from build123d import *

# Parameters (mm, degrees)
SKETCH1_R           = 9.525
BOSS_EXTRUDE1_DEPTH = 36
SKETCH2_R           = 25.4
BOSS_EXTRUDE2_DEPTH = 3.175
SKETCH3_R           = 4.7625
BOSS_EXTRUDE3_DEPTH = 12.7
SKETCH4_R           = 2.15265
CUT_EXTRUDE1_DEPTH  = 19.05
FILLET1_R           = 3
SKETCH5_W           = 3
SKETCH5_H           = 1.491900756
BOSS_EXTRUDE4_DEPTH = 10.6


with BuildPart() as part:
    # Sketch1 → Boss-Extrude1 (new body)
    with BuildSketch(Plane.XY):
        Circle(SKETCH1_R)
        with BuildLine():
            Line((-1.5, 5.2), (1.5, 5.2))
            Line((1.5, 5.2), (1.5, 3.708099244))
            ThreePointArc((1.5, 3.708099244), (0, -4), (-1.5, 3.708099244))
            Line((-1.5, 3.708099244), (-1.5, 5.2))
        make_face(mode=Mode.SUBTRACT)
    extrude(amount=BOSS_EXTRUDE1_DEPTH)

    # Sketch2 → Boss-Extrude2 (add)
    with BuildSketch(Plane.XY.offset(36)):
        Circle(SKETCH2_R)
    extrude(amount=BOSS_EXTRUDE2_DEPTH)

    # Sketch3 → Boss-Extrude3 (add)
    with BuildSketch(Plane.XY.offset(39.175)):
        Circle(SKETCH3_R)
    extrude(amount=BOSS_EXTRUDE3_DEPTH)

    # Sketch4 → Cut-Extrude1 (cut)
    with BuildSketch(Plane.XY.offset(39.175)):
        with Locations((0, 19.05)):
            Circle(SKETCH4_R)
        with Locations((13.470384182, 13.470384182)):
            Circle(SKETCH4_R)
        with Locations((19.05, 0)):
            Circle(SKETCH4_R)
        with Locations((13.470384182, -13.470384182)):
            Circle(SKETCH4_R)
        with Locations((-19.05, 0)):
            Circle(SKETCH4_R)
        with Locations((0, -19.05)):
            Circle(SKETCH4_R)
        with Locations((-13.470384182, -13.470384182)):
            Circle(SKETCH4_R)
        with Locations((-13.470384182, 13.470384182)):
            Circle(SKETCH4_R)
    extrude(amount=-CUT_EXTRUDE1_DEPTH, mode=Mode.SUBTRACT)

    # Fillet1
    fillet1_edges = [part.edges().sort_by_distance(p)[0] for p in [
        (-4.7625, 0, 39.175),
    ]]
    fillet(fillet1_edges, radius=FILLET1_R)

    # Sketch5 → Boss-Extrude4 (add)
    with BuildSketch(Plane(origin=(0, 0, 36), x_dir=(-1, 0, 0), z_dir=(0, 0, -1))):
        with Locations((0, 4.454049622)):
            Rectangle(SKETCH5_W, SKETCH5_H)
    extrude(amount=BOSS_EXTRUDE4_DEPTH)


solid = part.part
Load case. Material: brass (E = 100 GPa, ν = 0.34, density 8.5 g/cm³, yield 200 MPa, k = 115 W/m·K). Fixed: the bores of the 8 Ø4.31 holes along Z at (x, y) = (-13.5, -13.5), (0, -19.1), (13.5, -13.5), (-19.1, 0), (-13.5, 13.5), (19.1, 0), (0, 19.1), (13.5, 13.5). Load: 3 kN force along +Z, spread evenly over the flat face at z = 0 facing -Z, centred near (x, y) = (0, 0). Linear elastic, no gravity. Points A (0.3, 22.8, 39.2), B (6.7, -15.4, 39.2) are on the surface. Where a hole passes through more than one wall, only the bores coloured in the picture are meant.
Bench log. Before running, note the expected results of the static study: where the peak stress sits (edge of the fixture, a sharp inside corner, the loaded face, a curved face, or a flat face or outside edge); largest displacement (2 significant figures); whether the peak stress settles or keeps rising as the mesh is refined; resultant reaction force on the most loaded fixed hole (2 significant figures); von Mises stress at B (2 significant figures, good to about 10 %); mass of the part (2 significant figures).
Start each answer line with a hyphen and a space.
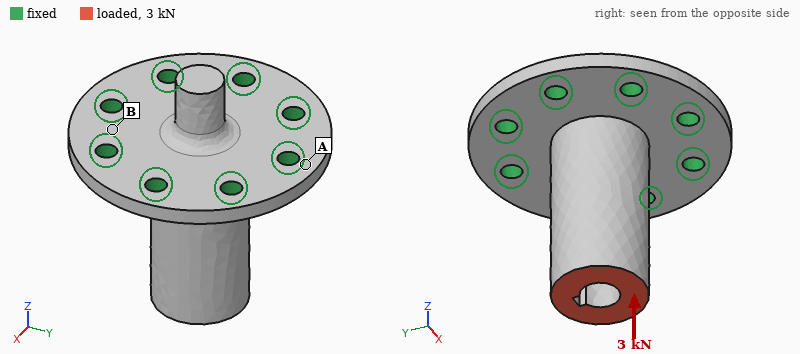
- edge of the fixture
- 19 µm
- keeps rising
- 410 N
- 34 MPa
- 130 g
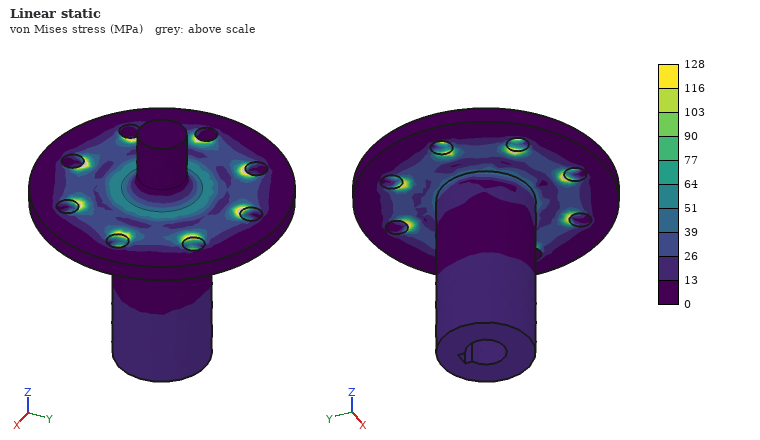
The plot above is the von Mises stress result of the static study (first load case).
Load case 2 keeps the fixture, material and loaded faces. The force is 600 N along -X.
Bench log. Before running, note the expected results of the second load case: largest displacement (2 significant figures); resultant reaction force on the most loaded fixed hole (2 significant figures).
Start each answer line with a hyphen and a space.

- 62 µm
- 420 N
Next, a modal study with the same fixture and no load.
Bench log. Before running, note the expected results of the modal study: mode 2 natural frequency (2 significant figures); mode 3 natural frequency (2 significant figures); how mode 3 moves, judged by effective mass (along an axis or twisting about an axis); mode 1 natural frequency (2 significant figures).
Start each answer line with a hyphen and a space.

- 3200 Hz
- 7400 Hz
- along Z
- 3200 Hz
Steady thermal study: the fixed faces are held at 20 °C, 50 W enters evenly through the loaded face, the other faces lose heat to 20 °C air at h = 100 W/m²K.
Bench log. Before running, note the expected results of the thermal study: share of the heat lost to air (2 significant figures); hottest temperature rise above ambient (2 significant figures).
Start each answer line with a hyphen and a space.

- 29 %
- 71 K
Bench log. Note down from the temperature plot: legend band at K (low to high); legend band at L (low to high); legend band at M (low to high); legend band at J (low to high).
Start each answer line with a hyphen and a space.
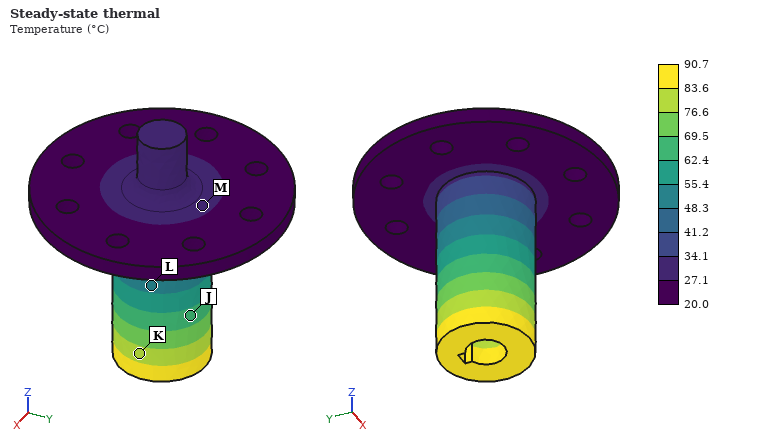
- 76.6 to 83.6 °C
- 48.3 to 55.4 °C
- 27.1 to 34.1 °C
- 62.4 to 69.5 °C
